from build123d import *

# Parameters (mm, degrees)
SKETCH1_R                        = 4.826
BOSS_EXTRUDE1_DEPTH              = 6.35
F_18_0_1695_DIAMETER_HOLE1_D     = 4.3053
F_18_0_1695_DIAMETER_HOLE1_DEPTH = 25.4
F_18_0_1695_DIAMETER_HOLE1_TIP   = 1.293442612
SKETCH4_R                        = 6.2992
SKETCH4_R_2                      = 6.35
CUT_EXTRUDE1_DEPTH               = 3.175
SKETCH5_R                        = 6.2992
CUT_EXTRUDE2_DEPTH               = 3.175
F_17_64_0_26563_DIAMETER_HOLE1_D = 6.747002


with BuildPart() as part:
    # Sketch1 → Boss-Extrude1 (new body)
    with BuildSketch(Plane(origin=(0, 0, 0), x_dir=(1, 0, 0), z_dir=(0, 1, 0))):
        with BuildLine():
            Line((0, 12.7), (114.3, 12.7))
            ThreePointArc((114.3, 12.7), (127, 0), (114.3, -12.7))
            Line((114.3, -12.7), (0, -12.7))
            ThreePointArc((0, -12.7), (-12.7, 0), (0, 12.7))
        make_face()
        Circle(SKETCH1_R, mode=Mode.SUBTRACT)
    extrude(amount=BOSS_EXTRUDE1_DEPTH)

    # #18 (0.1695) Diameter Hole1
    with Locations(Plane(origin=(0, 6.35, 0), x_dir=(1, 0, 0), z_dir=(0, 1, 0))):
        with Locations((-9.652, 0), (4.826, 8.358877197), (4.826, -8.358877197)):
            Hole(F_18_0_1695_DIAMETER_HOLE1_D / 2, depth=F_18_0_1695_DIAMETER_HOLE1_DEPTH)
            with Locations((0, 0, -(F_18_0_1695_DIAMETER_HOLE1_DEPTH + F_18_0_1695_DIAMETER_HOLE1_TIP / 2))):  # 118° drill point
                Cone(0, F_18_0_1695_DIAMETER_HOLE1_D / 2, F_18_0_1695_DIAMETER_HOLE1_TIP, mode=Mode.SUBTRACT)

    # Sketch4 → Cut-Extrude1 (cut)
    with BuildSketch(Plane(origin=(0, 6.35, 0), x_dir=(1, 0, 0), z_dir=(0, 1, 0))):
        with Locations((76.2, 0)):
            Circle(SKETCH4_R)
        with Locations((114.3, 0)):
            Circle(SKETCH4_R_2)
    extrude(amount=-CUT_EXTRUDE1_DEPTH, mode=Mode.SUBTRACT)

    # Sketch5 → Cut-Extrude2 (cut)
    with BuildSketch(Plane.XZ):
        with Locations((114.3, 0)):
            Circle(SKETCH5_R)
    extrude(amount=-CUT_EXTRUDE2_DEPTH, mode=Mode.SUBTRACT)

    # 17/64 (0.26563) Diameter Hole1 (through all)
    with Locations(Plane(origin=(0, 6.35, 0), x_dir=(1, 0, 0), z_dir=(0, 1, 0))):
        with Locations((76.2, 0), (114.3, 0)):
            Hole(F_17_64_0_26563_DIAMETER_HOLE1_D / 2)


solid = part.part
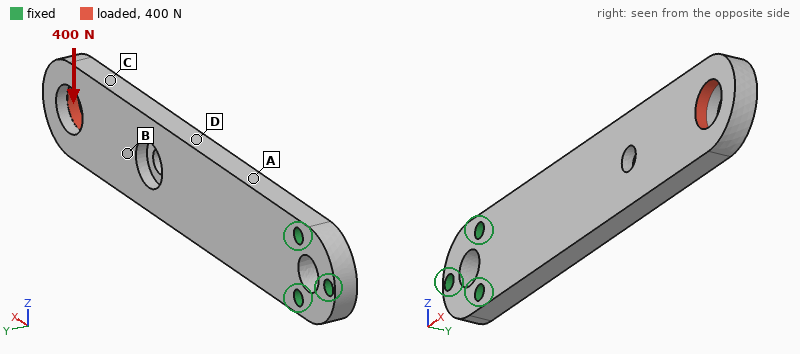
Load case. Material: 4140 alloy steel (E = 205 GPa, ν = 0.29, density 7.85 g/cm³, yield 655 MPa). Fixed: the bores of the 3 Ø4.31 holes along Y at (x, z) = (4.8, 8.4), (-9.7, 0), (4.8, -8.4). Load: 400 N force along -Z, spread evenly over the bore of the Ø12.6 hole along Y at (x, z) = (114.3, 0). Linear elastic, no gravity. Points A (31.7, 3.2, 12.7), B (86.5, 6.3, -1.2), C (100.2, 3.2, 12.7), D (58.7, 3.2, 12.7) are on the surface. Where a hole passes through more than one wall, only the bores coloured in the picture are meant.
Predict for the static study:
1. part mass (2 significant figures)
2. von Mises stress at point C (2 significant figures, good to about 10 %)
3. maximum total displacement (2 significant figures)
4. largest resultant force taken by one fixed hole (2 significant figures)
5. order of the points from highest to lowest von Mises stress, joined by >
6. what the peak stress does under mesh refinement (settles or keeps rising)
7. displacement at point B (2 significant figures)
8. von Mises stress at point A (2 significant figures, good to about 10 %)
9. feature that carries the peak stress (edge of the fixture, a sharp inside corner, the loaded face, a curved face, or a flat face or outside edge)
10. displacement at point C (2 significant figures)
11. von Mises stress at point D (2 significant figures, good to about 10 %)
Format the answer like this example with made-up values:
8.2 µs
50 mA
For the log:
150 g
10 MPa
0.12 mm
2.4 kN
A > D > C > B
keeps rising
0.063 mm
48 MPa
edge of the fixture
0.084 mm
33 MPa
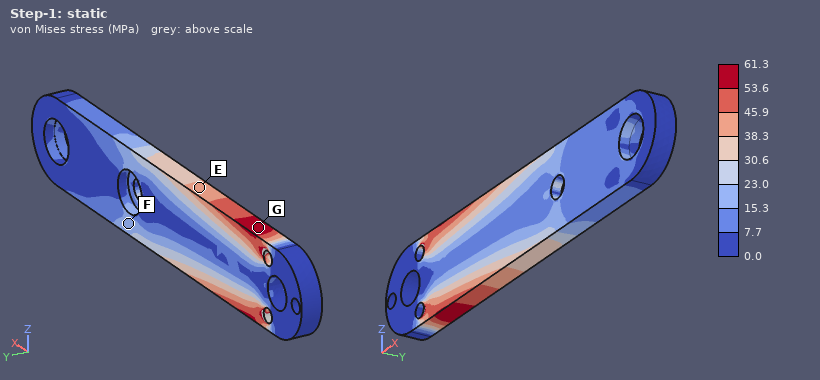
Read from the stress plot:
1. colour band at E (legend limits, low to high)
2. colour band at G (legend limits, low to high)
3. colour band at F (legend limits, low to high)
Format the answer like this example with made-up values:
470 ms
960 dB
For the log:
38.3 to 45.9 MPa
53.6 to 61.3 MPa
15.3 to 23.0 MPa
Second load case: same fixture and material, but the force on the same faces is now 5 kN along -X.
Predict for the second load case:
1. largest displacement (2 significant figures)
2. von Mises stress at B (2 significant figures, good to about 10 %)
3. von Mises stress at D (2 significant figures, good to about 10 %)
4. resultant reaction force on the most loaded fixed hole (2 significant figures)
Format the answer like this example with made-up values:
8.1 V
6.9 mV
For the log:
0.54 mm
19 MPa
35 MPa
2.5 kN
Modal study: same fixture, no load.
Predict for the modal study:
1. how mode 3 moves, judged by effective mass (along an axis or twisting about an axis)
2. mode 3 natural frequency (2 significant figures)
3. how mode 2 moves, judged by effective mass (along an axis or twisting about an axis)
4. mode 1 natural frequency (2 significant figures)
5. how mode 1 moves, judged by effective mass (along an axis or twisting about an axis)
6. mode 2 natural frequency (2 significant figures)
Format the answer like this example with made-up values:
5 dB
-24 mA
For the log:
along Y
2300 Hz
along Z
400 Hz
along Y
1500 Hz
